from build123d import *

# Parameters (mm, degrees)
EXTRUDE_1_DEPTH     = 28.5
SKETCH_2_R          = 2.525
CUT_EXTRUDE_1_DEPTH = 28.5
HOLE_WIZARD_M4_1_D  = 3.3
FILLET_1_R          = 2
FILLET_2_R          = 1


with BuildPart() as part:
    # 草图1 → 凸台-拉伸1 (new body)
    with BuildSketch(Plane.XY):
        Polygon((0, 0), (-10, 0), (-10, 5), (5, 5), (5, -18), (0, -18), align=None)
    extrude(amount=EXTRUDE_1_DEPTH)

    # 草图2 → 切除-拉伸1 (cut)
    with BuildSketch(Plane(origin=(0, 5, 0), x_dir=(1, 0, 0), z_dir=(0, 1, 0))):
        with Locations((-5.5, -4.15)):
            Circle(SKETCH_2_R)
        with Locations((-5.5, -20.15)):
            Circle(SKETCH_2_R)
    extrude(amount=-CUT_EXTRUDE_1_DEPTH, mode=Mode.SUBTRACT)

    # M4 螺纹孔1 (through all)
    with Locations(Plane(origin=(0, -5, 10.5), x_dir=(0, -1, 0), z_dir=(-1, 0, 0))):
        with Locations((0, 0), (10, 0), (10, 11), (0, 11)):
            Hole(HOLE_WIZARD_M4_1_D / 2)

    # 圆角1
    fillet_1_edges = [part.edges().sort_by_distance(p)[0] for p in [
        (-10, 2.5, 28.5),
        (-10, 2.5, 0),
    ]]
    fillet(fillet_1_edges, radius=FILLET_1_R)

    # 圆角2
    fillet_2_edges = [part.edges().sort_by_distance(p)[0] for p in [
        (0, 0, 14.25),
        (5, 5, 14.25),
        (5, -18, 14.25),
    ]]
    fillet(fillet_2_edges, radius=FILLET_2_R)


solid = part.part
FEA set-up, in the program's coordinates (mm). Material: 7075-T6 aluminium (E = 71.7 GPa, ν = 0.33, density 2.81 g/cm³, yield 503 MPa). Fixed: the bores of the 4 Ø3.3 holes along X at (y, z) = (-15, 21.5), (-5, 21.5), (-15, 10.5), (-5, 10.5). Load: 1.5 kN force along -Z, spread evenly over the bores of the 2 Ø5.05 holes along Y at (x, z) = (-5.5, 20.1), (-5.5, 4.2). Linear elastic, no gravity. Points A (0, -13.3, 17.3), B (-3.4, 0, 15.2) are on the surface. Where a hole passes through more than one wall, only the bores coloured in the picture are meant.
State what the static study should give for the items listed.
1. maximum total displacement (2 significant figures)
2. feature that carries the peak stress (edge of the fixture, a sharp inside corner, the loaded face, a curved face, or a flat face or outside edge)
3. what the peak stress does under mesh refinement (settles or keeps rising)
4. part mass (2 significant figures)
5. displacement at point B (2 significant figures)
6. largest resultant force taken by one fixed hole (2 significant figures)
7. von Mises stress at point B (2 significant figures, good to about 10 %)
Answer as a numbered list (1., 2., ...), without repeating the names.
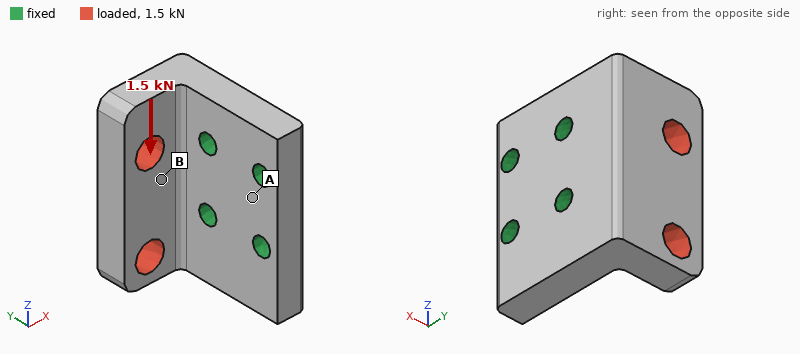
1. 30 µm
2. edge of the fixture
3. keeps rising
4. 12 g
5. 12 µm
6. 1.3 kN
7. 42 MPa
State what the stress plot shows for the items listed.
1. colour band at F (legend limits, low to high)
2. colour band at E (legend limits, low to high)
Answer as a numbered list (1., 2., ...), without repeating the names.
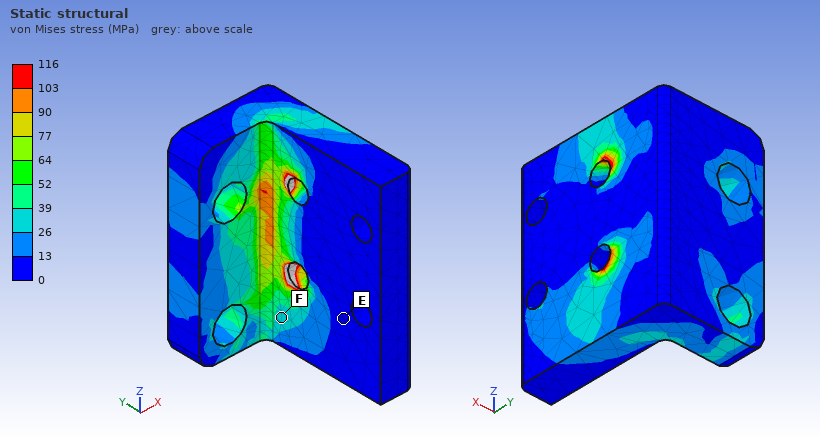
1. 26 to 39 MPa
2. 0 to 13 MPa
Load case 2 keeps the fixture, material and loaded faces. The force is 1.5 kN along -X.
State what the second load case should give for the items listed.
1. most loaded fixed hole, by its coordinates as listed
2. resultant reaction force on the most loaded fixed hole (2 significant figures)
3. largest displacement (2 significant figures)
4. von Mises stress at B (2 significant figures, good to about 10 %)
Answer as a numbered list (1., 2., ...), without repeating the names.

1. (-5, 10.5)
2. 1.2 kN
3. 44 µm
4. 22 MPa
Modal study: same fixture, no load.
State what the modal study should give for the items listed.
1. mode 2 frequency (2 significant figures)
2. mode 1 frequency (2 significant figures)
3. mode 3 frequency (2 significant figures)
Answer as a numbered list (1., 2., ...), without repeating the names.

1. 19 kHz
2. 14 kHz
3. 28 kHz
